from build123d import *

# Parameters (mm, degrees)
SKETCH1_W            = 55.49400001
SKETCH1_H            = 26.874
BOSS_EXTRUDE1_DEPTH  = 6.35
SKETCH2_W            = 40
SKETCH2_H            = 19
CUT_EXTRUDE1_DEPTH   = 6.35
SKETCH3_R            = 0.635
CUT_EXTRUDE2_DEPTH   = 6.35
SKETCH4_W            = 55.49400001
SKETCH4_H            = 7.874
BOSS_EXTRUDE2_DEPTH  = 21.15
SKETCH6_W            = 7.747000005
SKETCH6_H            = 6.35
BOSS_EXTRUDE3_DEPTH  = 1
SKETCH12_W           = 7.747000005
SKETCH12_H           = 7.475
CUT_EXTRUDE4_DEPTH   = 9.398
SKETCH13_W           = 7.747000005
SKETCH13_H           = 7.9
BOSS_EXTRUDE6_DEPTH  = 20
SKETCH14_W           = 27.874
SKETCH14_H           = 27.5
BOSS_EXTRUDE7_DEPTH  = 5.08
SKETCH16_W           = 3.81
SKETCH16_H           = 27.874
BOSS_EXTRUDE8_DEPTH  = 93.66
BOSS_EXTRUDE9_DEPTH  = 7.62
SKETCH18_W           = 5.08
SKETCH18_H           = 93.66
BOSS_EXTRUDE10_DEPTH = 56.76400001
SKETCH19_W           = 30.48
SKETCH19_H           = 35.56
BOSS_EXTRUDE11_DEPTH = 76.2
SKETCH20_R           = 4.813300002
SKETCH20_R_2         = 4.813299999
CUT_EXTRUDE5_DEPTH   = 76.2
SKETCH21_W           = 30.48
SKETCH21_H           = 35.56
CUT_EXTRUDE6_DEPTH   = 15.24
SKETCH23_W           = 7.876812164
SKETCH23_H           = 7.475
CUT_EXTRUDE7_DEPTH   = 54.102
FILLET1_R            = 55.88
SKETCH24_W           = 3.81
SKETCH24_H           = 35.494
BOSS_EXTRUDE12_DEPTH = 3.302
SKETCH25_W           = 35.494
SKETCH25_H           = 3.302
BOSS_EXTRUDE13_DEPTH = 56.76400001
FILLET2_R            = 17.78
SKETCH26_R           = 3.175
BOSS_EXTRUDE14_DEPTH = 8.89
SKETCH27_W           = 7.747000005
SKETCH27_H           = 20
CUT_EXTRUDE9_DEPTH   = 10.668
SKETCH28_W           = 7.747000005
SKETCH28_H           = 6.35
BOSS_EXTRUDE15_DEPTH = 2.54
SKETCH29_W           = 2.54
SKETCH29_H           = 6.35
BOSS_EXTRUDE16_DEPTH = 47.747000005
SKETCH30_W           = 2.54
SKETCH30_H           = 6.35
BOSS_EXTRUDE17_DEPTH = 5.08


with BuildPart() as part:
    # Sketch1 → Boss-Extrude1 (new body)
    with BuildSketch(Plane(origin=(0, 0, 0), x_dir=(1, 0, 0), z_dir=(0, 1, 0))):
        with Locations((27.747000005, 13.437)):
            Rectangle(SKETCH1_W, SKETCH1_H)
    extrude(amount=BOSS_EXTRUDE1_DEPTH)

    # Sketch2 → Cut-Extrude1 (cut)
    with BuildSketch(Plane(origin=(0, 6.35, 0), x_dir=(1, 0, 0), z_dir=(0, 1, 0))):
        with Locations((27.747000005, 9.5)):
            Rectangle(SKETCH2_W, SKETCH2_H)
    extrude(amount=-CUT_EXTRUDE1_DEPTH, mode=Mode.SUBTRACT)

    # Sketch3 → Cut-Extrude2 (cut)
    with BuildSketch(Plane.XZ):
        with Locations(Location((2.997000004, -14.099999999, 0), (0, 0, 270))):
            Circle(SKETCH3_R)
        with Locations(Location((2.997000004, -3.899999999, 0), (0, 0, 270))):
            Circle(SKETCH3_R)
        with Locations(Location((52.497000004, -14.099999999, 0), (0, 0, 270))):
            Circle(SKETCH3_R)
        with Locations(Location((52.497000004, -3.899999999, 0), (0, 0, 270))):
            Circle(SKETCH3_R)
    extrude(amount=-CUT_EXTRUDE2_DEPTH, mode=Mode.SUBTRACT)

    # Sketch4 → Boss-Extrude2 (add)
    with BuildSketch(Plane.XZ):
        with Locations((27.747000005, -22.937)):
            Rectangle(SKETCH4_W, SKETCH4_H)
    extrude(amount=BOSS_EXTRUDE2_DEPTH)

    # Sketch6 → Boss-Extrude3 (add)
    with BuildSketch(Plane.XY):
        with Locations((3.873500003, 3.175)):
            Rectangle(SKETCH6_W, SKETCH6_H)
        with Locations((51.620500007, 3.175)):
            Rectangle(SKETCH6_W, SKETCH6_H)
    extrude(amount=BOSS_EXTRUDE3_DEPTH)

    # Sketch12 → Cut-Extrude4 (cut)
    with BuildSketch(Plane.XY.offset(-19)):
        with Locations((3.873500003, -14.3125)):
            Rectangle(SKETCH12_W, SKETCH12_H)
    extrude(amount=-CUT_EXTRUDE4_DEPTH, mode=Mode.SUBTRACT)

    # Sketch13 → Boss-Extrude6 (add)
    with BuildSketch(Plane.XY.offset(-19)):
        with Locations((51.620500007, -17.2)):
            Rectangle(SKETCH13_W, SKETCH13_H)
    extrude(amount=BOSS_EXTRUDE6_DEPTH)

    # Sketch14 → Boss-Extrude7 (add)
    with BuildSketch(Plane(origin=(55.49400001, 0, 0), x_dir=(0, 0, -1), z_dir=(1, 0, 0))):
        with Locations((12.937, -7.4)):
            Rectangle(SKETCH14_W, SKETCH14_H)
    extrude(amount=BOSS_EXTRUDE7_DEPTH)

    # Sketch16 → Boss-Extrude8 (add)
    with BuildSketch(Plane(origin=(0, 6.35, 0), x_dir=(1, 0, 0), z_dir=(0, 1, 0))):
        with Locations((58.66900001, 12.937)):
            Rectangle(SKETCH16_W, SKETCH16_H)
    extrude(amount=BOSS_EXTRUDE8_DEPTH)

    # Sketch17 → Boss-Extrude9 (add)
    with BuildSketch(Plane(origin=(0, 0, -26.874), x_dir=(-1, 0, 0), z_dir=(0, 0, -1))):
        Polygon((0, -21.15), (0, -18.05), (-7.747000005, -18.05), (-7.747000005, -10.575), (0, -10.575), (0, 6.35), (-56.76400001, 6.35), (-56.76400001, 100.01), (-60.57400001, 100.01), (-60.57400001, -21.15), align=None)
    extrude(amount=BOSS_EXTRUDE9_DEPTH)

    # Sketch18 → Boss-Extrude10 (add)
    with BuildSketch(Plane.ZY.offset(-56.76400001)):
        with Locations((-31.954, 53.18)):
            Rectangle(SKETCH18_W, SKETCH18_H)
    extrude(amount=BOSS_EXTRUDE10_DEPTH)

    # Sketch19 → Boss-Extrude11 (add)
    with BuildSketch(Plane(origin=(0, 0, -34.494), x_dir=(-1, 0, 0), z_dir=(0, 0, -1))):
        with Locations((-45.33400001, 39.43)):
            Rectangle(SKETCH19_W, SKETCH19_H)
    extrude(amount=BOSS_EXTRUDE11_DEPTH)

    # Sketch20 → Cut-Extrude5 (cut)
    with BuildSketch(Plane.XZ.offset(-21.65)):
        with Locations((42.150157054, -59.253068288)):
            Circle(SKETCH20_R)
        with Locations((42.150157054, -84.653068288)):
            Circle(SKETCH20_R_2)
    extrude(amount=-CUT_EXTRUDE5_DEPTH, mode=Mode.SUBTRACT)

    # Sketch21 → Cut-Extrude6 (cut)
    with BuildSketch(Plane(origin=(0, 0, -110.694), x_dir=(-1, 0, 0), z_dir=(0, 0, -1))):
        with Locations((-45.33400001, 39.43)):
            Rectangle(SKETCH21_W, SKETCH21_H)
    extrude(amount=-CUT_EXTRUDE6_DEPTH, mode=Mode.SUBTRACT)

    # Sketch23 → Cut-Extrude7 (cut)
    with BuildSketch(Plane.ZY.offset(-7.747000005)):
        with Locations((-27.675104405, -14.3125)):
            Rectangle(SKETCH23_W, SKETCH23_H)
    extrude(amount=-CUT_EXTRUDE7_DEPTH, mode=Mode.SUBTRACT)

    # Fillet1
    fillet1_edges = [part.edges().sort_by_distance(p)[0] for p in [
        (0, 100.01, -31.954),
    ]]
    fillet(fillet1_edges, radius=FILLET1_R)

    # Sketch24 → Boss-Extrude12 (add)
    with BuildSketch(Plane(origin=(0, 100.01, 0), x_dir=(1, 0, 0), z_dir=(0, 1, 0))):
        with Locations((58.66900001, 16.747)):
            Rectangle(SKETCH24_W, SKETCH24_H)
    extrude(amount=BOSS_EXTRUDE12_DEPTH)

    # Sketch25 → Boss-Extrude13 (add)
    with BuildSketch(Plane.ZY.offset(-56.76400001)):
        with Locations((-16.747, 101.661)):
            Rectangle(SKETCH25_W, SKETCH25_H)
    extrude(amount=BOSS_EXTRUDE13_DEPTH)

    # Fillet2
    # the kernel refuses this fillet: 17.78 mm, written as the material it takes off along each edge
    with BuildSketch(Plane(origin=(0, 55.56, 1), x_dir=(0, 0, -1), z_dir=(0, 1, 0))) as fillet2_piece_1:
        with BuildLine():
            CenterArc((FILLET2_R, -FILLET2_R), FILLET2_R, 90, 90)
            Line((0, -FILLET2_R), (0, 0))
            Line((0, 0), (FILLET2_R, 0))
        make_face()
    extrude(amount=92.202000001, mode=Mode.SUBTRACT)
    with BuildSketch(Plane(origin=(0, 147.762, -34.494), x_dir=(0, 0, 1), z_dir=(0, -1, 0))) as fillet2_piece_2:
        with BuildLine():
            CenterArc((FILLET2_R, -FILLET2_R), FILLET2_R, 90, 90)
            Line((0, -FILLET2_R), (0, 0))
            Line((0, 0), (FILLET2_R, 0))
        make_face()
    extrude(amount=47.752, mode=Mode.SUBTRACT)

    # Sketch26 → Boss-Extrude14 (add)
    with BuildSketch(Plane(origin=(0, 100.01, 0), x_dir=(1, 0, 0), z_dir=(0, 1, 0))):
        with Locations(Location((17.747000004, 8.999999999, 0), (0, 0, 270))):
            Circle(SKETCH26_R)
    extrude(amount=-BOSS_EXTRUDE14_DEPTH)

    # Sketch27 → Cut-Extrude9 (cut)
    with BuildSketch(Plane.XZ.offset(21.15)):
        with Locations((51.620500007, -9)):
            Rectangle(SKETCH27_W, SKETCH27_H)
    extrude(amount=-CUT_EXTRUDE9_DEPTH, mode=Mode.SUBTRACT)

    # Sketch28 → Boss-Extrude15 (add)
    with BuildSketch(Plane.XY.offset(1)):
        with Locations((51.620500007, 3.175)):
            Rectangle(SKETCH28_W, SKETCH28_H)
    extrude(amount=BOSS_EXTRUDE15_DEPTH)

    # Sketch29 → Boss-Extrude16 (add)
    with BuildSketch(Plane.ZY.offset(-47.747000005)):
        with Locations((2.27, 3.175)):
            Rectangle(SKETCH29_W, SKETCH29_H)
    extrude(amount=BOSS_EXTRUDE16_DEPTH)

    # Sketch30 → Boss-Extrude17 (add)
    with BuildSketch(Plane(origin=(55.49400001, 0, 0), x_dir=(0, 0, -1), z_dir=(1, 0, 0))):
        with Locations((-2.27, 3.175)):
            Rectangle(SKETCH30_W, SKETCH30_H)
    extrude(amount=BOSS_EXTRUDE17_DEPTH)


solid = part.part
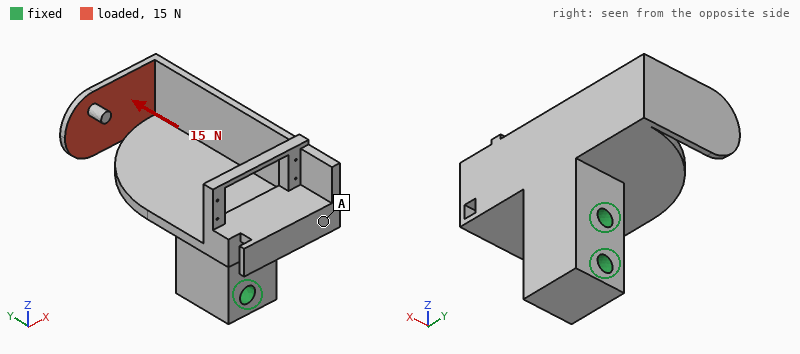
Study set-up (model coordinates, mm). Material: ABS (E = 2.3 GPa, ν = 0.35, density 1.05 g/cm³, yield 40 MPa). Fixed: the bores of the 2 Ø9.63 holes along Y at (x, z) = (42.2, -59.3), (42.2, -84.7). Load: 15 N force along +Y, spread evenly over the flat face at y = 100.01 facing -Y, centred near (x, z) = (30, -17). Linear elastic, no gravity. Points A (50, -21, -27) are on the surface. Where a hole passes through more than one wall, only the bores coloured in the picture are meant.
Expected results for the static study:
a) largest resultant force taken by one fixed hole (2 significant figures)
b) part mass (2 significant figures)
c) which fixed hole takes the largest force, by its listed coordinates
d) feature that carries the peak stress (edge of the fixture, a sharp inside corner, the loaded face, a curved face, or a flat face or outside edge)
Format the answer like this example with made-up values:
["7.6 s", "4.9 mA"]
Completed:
["18 N", "140 g", "(42.2, -59.3)", "a curved face"]
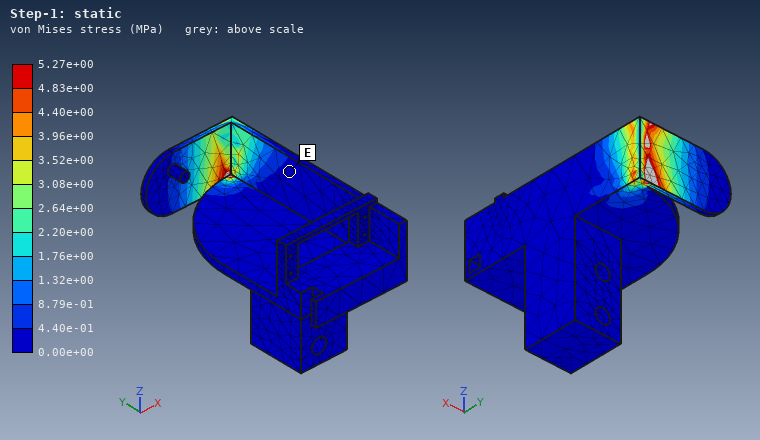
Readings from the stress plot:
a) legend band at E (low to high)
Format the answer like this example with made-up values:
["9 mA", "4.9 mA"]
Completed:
["0.00e+00 to 4.40e-01 MPa"]
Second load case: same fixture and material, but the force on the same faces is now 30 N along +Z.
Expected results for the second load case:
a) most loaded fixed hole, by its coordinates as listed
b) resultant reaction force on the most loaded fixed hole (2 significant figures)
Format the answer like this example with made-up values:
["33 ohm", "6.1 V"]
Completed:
["(42.2, -59.3)", "32 N"]
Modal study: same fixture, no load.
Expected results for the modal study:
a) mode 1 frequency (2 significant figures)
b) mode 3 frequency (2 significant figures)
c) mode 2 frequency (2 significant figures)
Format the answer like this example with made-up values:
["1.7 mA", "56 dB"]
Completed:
["210 Hz", "550 Hz", "280 Hz"]
